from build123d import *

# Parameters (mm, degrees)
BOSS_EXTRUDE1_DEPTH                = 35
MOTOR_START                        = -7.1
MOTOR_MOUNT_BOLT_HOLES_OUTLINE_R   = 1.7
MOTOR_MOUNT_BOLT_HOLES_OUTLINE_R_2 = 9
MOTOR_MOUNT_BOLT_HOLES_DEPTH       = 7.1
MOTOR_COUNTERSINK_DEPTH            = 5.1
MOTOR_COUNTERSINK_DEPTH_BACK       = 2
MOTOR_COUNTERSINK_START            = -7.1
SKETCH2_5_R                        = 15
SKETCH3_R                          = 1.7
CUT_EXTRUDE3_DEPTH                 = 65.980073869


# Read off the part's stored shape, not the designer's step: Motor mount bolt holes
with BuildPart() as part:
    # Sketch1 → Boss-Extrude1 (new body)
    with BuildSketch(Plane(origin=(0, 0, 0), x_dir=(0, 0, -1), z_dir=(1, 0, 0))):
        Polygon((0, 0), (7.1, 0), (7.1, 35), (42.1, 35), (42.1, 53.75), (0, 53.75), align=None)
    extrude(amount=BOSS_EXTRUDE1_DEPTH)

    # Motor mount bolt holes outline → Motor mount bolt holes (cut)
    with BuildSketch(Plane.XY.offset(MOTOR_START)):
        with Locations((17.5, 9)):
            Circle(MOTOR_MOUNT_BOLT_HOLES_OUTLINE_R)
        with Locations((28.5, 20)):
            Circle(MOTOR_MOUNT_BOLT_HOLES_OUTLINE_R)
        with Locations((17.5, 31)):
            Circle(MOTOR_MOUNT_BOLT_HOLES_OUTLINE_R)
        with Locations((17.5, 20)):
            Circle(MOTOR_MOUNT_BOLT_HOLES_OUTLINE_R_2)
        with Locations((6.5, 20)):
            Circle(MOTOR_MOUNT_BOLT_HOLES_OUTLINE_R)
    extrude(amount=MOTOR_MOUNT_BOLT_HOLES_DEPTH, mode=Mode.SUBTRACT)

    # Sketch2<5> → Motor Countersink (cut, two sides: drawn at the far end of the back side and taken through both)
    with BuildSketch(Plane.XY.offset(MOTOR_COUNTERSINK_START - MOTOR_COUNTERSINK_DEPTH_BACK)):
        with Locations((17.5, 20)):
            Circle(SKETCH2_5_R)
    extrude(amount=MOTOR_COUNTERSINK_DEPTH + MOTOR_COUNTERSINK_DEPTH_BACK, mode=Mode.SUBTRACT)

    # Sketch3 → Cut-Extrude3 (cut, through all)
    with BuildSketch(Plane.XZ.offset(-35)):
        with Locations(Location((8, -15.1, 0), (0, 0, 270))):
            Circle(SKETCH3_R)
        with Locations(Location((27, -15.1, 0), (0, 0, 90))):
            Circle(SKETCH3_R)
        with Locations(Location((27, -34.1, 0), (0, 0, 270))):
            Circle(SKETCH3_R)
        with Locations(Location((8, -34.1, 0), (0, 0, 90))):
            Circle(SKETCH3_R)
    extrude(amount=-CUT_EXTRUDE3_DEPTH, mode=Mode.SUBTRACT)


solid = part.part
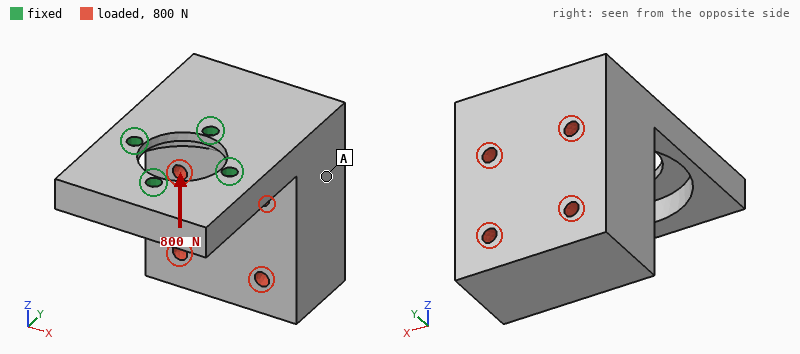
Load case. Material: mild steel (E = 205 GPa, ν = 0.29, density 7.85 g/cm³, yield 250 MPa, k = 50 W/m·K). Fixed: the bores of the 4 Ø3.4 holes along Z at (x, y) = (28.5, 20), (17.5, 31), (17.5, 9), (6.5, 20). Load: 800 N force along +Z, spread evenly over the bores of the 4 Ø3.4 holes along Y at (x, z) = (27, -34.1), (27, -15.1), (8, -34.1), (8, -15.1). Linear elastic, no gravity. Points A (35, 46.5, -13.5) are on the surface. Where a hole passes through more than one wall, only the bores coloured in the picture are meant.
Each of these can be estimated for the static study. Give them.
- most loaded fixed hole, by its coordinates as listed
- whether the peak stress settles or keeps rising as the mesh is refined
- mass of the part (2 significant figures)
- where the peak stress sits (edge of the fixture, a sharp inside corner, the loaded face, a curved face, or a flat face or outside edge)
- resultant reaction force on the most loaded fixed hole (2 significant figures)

(17.5, 31)
keeps rising
250 g
edge of the fixture
1.4 kN
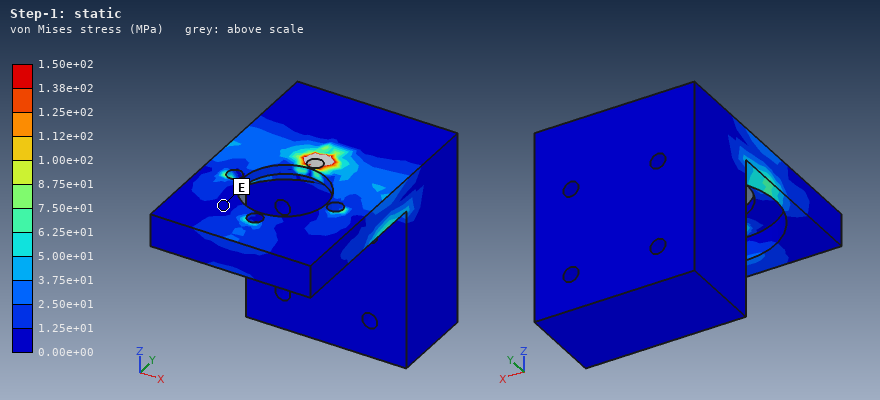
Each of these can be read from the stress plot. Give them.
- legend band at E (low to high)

0.00e+00 to 1.25e+01 MPa
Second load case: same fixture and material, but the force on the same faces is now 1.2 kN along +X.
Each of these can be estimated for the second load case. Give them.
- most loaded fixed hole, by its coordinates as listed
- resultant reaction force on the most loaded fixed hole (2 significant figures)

(17.5, 31)
1.3 kN
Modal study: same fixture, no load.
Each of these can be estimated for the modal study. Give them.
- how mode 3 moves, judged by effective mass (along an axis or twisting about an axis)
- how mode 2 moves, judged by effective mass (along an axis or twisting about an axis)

along Z
along X
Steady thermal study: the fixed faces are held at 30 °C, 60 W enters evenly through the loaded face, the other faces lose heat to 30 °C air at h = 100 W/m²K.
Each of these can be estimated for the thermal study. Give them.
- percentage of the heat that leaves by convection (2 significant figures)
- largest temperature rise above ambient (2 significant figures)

65 %
73 K
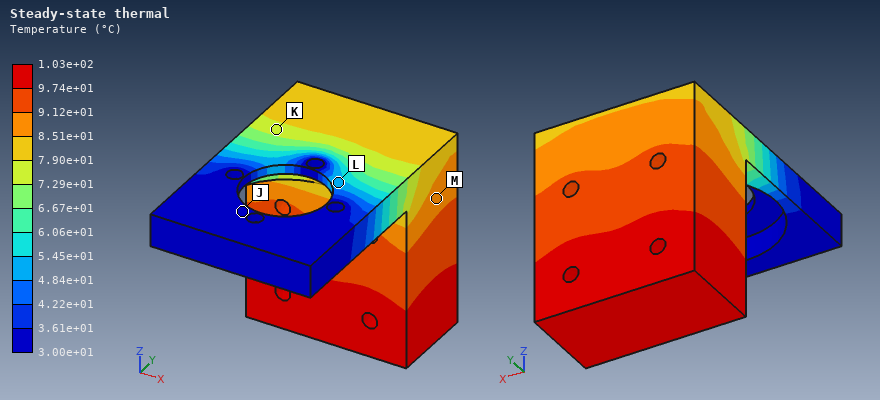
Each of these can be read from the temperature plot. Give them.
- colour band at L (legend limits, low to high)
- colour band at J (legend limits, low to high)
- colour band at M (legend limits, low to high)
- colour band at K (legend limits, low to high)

4.84e+01 to 5.45e+01 °C
3.00e+01 to 3.61e+01 °C
8.51e+01 to 9.12e+01 °C
7.29e+01 to 7.90e+01 °C
